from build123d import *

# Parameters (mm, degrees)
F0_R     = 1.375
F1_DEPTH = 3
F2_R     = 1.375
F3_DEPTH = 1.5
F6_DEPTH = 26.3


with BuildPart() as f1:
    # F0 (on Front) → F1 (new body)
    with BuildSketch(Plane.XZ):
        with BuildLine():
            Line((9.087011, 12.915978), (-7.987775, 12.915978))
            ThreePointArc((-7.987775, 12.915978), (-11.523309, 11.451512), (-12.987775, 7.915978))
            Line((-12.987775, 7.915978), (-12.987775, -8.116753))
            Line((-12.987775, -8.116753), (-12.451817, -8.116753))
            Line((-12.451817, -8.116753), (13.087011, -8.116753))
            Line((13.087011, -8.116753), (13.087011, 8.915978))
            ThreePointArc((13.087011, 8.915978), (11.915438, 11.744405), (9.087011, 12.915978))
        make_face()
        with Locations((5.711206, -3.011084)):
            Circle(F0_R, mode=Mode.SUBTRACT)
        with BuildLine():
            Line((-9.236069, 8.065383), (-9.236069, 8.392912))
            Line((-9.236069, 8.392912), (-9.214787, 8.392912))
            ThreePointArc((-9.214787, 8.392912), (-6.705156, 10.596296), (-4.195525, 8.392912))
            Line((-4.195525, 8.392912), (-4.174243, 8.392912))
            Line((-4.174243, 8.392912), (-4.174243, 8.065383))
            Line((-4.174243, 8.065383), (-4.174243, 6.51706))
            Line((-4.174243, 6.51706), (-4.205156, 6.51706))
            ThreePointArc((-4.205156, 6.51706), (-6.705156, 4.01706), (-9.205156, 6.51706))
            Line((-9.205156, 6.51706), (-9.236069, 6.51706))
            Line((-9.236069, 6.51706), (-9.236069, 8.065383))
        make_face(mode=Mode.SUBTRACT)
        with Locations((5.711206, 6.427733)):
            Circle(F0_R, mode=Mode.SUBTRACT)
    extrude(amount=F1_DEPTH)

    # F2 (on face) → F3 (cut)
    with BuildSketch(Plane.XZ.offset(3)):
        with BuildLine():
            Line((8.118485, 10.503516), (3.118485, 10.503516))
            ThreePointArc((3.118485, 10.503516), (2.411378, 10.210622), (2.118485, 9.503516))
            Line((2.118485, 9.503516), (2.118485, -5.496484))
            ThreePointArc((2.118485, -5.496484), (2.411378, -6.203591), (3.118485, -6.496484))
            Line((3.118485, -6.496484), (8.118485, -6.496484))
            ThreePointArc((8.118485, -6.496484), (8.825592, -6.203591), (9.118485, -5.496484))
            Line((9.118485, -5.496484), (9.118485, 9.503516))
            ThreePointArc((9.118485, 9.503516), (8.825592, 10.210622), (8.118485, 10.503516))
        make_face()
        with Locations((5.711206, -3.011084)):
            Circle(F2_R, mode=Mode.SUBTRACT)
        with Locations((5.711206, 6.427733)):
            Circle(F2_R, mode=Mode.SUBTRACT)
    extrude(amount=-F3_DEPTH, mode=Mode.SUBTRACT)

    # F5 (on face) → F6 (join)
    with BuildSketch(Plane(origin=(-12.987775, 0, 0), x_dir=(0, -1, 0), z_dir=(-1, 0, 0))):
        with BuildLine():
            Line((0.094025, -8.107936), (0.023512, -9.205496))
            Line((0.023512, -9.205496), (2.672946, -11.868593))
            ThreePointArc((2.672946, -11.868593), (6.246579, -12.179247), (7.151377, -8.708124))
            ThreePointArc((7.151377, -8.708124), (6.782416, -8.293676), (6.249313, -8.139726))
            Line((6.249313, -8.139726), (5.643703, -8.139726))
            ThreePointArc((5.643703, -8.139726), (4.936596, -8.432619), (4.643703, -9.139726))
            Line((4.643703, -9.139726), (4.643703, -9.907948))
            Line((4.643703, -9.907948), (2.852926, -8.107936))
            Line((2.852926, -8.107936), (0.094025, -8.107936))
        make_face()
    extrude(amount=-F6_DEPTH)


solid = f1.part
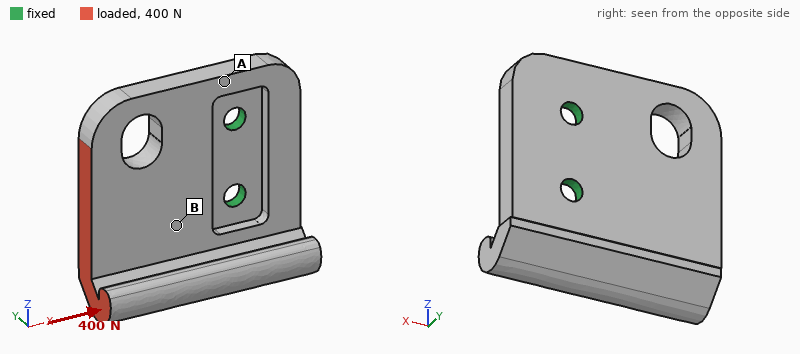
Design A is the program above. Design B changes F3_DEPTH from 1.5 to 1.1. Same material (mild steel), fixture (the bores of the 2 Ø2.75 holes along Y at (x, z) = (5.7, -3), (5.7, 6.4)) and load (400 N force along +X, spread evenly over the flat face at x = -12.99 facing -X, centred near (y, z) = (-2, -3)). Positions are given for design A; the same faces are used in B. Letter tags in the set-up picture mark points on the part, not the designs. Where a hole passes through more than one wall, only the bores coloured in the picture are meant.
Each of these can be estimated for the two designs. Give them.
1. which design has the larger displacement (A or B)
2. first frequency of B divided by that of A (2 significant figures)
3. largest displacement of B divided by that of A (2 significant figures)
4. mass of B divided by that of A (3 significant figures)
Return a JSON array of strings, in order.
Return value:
["A", "1.2", "0.62", "1.02"]
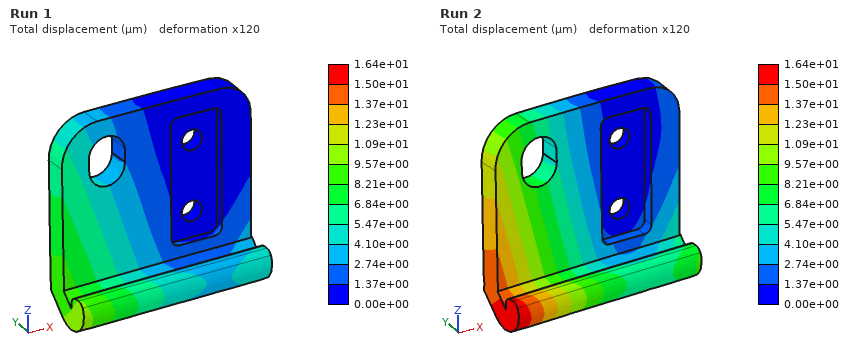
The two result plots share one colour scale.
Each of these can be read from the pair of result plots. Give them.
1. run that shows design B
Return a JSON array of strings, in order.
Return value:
["Run 1"]
